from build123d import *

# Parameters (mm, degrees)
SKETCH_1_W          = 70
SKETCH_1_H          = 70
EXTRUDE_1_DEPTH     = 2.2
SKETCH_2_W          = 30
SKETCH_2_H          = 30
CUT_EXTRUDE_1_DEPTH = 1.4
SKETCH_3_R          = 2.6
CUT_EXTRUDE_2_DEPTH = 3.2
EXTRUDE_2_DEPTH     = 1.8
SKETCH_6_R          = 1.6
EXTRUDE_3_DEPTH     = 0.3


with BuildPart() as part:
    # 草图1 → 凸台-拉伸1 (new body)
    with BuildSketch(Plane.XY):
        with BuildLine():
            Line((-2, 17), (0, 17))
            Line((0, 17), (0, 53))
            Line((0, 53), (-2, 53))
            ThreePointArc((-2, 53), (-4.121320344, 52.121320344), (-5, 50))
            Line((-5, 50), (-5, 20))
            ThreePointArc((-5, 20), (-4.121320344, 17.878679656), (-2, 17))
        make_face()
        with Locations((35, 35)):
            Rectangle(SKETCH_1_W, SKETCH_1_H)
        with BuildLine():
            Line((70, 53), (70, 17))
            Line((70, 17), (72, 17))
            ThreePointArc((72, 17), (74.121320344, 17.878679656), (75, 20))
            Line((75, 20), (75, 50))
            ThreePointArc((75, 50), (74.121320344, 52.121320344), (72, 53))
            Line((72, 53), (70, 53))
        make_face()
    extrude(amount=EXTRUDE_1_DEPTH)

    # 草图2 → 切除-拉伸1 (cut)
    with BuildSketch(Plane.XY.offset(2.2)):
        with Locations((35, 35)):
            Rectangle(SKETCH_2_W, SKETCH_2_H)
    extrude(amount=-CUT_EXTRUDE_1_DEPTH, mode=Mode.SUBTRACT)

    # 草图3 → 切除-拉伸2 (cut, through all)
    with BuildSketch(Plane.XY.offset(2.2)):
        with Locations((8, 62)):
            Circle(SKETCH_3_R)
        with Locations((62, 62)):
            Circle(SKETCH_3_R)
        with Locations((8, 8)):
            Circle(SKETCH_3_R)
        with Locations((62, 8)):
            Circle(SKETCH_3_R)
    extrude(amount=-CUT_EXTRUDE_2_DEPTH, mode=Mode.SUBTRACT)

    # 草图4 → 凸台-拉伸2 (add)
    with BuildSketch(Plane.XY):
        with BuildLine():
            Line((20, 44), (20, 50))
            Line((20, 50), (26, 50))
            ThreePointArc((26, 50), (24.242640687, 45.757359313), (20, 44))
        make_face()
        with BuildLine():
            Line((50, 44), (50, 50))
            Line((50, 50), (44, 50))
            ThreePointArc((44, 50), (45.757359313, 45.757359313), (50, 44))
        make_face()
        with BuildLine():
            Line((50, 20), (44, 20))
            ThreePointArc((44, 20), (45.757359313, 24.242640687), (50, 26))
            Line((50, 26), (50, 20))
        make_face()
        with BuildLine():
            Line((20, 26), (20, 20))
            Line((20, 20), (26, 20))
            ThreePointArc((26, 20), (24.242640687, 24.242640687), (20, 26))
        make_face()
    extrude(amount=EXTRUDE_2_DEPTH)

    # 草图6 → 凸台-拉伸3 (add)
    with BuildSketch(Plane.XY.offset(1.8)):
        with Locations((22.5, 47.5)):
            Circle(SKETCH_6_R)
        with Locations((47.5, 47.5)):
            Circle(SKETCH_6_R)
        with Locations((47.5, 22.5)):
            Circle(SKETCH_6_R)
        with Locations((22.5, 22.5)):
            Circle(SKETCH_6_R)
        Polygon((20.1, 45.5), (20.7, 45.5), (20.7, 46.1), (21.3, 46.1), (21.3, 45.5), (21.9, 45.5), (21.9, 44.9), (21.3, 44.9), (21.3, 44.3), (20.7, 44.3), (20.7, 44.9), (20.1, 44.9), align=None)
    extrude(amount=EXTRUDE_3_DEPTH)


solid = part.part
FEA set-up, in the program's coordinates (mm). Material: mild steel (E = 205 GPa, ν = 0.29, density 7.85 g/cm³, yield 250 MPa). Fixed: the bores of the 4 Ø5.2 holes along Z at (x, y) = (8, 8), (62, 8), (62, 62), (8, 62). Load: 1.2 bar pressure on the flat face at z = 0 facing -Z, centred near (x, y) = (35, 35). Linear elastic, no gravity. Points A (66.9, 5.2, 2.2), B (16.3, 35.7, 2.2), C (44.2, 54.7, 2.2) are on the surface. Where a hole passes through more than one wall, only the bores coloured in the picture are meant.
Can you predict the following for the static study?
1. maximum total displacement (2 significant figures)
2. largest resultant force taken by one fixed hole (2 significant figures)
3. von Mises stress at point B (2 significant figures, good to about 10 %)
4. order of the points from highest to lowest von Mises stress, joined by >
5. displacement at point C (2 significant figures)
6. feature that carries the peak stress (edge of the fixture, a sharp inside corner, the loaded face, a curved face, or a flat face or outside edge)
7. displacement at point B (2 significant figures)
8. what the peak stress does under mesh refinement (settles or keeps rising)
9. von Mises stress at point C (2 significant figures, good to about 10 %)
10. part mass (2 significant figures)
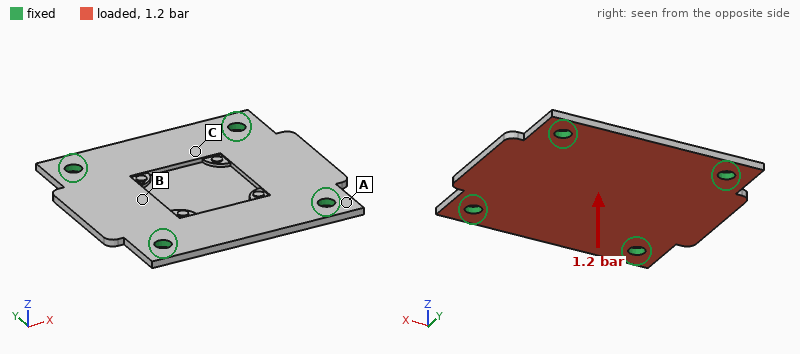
52 µm
180 N
29 MPa
B > C > A
20 µm
edge of the fixture
26 µm
keeps rising
18 MPa
80 g
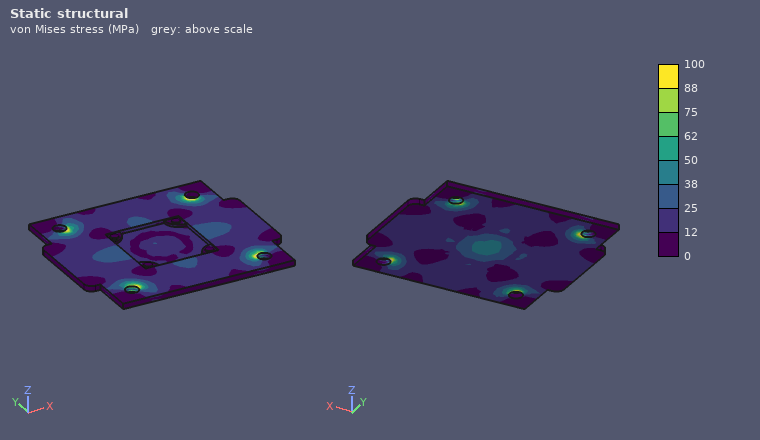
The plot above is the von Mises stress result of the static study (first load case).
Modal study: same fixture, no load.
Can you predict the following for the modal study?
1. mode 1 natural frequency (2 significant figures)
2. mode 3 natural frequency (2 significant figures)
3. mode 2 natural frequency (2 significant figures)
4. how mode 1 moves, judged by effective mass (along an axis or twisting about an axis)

3200 Hz
4100 Hz
4000 Hz
along Z
